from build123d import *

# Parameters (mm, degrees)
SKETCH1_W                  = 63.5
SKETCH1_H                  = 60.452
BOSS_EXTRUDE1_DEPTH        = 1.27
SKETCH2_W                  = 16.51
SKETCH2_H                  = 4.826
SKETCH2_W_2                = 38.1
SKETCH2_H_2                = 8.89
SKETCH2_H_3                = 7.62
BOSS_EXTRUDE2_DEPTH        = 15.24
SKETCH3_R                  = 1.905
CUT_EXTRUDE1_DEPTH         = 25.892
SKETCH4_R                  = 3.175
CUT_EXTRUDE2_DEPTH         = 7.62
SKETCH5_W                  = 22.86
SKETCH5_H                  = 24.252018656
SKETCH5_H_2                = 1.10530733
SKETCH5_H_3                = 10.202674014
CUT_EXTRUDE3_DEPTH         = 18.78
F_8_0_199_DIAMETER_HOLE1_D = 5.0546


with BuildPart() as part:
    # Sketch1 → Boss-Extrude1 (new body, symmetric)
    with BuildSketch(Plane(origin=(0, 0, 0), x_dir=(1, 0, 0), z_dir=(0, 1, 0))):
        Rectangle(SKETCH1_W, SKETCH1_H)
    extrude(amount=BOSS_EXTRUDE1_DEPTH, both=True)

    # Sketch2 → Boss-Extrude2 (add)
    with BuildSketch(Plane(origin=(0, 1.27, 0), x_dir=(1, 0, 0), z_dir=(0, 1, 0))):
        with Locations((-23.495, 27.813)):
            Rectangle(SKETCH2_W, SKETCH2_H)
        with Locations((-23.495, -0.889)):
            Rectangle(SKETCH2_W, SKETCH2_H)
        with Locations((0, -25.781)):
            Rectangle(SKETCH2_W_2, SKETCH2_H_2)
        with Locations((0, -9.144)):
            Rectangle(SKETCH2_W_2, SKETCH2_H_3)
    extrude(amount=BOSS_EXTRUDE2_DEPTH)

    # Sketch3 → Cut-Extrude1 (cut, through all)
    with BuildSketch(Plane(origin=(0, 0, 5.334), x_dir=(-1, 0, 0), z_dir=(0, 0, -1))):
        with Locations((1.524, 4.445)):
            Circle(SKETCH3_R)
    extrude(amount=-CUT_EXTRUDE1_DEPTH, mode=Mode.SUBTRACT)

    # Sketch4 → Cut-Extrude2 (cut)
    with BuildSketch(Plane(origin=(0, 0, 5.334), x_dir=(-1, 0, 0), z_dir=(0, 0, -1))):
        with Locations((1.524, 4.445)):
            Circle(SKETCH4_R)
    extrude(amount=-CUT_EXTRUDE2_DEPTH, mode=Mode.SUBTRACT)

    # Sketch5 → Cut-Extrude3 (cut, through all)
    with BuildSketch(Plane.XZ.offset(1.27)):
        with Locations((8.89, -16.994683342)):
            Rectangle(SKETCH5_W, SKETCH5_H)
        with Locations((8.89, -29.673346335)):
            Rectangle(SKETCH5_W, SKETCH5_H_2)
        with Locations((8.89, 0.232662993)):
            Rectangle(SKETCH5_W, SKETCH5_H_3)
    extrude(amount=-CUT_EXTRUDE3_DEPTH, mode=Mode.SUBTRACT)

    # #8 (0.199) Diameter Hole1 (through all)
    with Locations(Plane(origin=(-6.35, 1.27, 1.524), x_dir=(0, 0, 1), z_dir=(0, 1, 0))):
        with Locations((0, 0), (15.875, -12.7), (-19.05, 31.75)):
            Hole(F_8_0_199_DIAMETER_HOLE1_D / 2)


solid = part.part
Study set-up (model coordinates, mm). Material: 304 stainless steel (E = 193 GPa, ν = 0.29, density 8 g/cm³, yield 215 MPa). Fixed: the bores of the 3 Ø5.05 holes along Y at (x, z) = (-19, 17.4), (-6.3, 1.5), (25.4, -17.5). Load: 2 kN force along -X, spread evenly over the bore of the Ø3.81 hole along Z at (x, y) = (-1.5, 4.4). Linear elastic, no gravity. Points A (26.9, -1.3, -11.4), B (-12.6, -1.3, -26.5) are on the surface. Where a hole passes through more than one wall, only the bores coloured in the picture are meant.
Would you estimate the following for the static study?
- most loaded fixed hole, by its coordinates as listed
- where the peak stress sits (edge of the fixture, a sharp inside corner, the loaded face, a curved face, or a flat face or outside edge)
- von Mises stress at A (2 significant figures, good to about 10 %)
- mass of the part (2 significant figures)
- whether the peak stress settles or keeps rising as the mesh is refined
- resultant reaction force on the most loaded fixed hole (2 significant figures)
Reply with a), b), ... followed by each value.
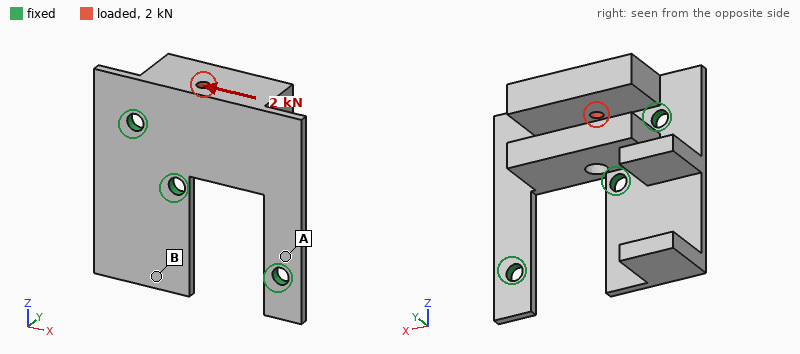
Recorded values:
a) (-19, 17.4)
b) edge of the fixture
c) 45 MPa
d) 150 g
e) keeps rising
f) 1.8 kN
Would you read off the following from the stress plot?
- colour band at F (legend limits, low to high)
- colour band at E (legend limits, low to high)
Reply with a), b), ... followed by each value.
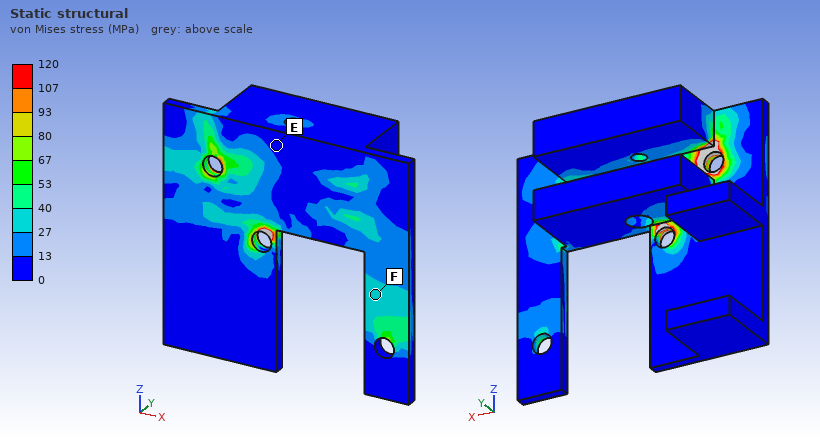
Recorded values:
a) 27 to 40 MPa
b) 0 to 13 MPa
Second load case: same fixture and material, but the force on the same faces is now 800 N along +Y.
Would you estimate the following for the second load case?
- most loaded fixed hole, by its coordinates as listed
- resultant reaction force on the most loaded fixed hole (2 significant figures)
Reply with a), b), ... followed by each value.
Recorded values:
a) (-19, 17.4)
b) 630 N
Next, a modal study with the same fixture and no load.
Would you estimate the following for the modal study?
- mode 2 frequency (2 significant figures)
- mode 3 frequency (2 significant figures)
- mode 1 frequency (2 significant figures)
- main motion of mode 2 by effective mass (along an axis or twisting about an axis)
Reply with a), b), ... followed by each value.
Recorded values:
a) 1600 Hz
b) 2600 Hz
c) 1000 Hz
d) along Y
